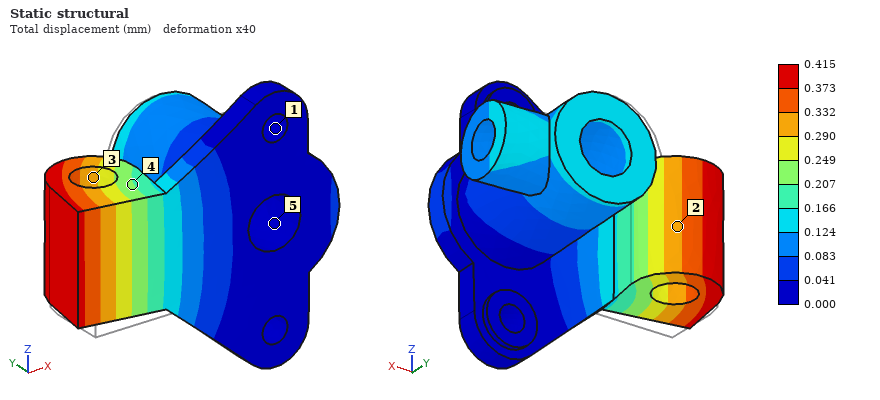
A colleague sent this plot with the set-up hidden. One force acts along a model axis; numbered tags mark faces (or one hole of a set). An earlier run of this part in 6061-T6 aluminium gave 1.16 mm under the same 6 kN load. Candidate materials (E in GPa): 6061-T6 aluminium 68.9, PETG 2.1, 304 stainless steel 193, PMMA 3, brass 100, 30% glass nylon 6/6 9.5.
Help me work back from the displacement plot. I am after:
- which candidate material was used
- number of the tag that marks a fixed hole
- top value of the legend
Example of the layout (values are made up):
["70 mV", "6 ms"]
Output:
["304 stainless steel", "1", "0.415 mm"]
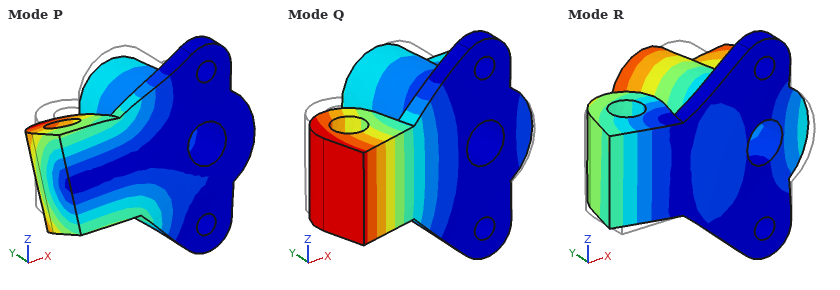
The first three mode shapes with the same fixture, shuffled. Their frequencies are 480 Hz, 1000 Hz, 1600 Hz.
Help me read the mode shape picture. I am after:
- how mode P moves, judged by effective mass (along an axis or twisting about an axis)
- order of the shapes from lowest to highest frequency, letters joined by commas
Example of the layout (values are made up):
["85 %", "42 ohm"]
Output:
["along Z", "Q, R, P"]
